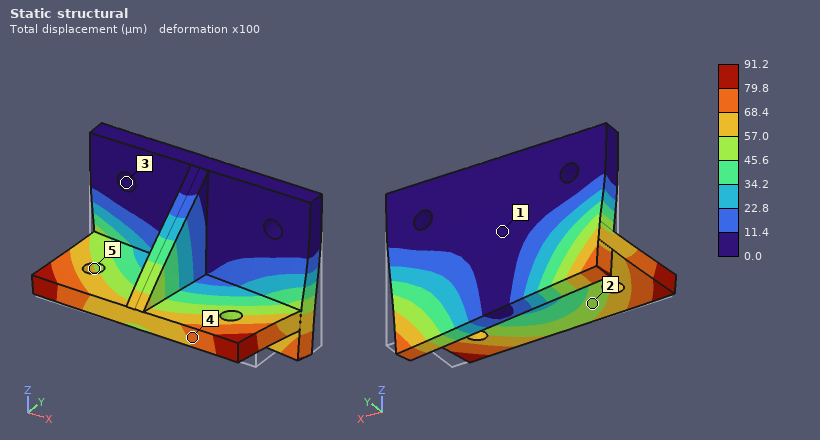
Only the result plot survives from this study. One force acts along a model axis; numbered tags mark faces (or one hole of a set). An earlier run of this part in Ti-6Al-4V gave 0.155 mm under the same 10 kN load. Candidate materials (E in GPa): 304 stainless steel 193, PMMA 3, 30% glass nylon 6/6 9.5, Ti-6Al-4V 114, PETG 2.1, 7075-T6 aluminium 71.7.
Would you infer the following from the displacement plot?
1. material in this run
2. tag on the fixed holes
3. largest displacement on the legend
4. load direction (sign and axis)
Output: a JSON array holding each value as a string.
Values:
["304 stainless steel", "3", "91.2 µm", "-X"]
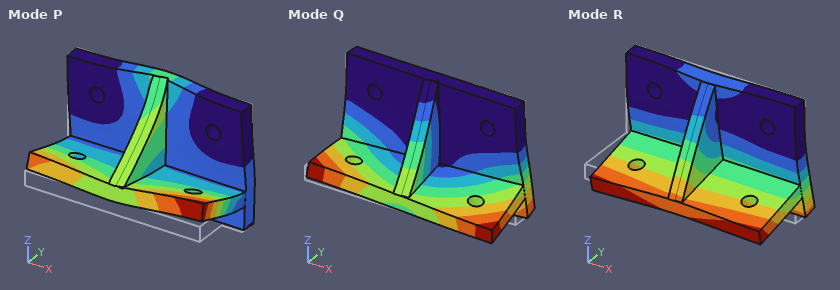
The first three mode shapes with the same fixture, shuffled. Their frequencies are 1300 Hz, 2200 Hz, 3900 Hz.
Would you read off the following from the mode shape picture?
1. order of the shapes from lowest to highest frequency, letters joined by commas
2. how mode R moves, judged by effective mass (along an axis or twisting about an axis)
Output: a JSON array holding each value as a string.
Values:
["R, Q, P", "along Y"]
